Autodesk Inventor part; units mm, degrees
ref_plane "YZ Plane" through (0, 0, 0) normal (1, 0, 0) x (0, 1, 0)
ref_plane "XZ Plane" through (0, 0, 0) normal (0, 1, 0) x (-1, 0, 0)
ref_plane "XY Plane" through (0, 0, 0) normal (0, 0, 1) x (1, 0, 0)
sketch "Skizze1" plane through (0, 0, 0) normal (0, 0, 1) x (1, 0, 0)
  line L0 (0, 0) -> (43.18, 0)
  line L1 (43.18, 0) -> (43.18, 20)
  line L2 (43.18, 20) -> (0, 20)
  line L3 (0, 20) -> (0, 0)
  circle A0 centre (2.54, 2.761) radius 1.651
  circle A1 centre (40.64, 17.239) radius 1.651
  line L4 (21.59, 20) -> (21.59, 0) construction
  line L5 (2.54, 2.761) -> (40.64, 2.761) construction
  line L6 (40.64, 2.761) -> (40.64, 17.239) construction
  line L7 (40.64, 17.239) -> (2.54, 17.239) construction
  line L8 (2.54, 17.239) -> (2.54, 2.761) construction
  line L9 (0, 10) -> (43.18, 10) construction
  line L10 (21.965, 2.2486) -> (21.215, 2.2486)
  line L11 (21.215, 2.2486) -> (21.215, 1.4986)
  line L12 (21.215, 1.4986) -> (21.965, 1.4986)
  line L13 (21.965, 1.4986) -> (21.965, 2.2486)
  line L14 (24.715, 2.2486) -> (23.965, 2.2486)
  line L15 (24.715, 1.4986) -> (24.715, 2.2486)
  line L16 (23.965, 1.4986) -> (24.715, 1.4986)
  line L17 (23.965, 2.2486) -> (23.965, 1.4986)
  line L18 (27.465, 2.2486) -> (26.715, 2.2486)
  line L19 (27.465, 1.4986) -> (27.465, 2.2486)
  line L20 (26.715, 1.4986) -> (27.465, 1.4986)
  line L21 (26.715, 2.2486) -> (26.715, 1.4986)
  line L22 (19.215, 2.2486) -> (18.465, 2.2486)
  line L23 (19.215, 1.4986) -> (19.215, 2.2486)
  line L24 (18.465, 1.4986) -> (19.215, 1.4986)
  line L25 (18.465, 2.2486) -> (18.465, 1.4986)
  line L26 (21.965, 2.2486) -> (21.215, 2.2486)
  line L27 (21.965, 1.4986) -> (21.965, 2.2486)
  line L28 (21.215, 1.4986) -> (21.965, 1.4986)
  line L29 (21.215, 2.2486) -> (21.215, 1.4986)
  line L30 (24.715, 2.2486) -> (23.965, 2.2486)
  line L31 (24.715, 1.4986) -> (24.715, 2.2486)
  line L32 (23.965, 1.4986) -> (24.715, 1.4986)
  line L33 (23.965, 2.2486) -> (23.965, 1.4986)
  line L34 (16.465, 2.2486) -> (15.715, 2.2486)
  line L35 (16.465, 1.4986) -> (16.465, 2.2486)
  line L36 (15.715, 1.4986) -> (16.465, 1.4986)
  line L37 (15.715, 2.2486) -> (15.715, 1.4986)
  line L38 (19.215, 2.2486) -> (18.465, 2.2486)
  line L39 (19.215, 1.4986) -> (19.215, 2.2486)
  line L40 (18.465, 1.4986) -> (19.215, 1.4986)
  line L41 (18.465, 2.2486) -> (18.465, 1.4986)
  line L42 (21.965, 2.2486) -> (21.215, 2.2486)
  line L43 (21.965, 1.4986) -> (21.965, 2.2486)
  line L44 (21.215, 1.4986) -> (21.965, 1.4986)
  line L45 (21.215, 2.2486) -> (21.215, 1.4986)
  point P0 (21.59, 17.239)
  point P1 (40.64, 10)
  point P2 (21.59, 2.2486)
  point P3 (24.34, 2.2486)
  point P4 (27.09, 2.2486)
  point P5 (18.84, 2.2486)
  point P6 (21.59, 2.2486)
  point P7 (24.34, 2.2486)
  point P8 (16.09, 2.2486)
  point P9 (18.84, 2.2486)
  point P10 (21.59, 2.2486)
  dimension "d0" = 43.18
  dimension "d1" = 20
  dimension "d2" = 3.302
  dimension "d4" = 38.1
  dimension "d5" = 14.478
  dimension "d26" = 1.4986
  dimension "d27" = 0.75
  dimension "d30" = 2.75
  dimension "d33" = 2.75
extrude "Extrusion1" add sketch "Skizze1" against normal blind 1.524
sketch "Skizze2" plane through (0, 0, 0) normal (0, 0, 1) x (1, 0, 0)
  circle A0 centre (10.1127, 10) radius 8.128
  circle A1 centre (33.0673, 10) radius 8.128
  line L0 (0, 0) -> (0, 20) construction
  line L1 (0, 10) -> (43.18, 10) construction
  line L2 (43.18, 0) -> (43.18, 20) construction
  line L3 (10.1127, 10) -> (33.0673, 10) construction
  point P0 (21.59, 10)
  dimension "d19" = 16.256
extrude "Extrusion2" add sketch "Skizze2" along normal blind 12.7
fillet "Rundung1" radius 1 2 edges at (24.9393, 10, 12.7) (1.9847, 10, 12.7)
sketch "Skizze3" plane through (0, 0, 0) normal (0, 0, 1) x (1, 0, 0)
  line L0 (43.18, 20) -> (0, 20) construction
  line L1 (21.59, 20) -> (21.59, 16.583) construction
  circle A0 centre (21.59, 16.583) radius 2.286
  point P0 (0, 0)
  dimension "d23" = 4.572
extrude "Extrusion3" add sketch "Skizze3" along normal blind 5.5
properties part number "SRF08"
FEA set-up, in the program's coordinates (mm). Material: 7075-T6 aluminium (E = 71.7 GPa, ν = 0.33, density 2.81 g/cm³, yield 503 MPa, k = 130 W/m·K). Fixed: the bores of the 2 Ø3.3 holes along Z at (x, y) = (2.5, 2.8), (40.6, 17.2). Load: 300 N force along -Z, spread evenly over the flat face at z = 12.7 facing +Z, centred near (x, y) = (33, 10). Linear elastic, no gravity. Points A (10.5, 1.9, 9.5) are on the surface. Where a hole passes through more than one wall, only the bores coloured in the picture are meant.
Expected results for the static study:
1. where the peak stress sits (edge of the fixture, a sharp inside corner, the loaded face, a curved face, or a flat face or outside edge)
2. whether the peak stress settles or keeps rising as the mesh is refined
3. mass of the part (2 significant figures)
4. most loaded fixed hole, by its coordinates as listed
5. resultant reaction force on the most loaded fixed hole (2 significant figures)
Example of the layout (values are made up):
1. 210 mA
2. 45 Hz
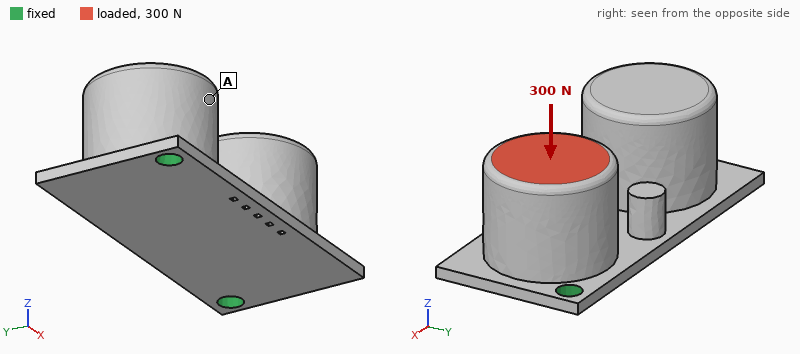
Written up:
1. edge of the fixture
2. keeps rising
3. 19 g
4. (40.6, 17.2)
5. 230 N
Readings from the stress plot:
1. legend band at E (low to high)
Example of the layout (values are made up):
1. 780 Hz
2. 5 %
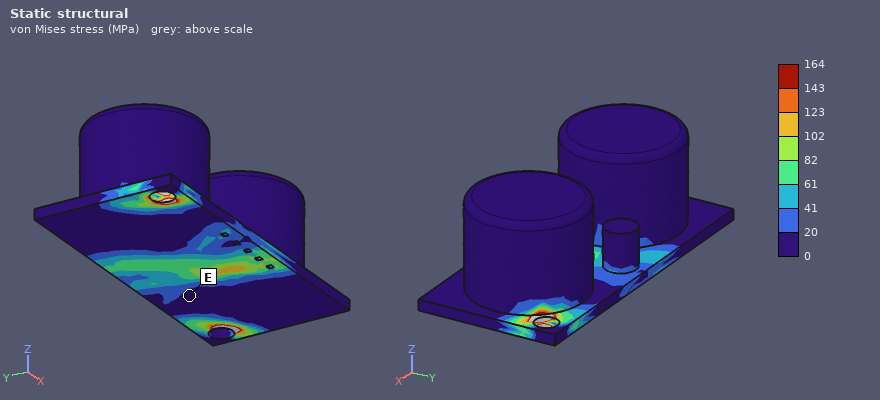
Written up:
1. 0 to 20 MPa
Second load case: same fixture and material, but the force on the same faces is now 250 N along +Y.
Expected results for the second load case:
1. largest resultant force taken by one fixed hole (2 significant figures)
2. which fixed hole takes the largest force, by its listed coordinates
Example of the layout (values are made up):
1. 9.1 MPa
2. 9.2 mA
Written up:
1. 220 N
2. (40.6, 17.2)
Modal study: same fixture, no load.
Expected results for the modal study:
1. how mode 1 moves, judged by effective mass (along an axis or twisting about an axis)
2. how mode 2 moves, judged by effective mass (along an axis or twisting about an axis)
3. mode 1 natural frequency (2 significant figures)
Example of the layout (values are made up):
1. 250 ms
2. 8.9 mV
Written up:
1. along Z
2. along Y
3. 2100 Hz
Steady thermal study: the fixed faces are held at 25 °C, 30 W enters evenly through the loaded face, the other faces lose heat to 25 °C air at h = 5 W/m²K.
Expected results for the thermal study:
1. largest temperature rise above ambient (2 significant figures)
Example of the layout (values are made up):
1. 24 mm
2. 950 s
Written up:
1. 58 K
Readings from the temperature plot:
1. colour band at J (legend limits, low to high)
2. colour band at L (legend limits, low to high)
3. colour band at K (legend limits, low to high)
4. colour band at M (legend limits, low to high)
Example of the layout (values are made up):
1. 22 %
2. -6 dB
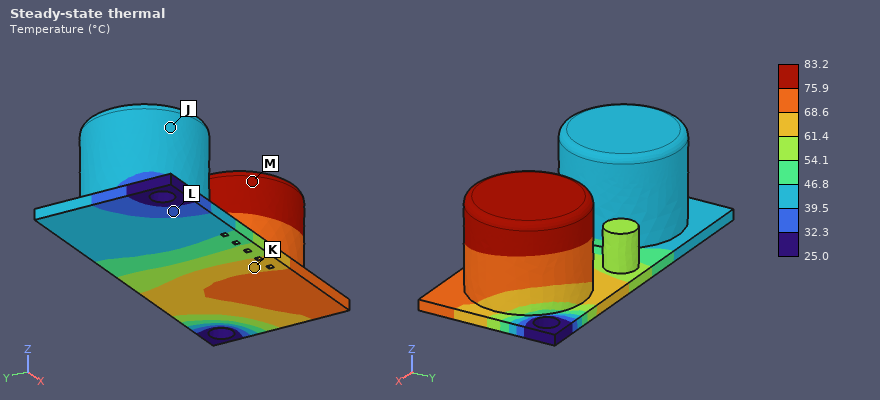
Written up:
1. 39.5 to 46.8 °C
2. 32.3 to 39.5 °C
3. 61.4 to 68.6 °C
4. 75.9 to 83.2 °C
